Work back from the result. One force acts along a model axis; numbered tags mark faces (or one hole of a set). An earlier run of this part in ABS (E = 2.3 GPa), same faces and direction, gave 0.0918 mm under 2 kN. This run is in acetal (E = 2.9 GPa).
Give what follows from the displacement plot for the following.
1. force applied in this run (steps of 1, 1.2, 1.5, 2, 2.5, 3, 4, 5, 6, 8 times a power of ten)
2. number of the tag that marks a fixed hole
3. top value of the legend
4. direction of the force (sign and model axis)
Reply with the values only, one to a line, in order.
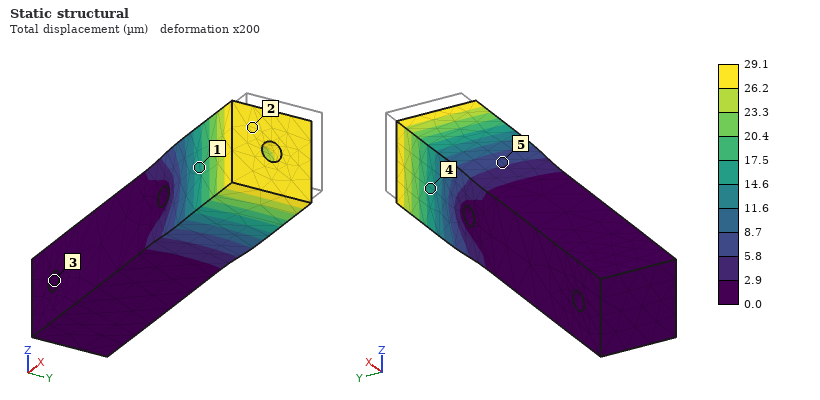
800 N
3
29.1 µm
-X
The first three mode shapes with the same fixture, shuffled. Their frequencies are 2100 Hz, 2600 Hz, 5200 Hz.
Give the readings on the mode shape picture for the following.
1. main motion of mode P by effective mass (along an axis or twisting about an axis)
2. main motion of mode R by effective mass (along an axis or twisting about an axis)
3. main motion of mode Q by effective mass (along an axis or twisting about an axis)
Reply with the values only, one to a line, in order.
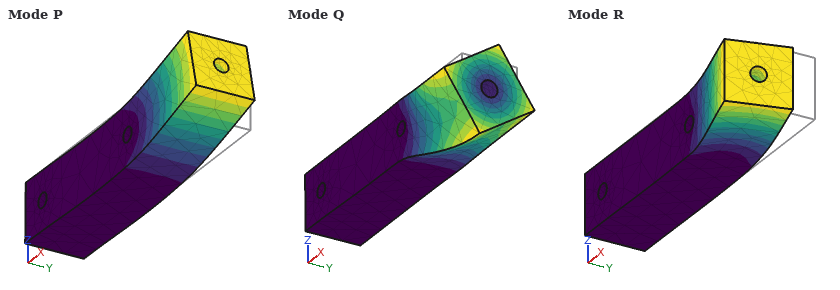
along Z
along Y
twisting about X
